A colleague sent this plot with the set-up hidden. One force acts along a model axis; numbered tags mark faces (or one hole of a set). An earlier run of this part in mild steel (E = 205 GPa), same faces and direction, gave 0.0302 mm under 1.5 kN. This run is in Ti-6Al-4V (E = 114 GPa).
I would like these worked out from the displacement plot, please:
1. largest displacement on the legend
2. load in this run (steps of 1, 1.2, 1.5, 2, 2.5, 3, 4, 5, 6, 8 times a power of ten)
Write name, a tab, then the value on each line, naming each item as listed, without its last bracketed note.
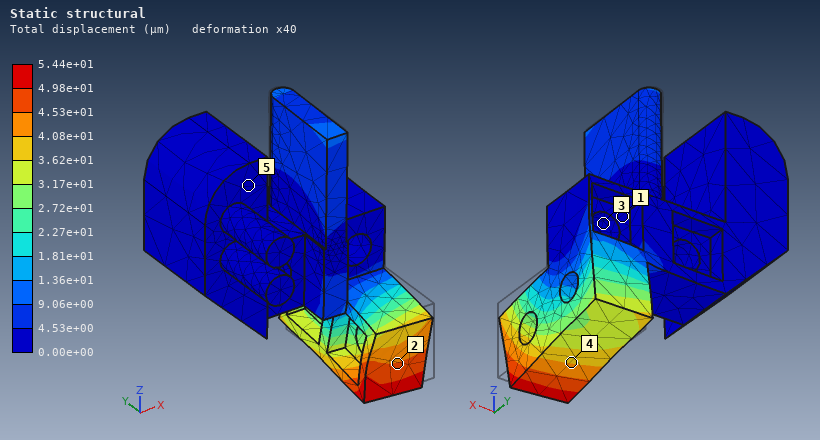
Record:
largest displacement on the legend	5.44e+01 µm
load in this run	1.5 kN
